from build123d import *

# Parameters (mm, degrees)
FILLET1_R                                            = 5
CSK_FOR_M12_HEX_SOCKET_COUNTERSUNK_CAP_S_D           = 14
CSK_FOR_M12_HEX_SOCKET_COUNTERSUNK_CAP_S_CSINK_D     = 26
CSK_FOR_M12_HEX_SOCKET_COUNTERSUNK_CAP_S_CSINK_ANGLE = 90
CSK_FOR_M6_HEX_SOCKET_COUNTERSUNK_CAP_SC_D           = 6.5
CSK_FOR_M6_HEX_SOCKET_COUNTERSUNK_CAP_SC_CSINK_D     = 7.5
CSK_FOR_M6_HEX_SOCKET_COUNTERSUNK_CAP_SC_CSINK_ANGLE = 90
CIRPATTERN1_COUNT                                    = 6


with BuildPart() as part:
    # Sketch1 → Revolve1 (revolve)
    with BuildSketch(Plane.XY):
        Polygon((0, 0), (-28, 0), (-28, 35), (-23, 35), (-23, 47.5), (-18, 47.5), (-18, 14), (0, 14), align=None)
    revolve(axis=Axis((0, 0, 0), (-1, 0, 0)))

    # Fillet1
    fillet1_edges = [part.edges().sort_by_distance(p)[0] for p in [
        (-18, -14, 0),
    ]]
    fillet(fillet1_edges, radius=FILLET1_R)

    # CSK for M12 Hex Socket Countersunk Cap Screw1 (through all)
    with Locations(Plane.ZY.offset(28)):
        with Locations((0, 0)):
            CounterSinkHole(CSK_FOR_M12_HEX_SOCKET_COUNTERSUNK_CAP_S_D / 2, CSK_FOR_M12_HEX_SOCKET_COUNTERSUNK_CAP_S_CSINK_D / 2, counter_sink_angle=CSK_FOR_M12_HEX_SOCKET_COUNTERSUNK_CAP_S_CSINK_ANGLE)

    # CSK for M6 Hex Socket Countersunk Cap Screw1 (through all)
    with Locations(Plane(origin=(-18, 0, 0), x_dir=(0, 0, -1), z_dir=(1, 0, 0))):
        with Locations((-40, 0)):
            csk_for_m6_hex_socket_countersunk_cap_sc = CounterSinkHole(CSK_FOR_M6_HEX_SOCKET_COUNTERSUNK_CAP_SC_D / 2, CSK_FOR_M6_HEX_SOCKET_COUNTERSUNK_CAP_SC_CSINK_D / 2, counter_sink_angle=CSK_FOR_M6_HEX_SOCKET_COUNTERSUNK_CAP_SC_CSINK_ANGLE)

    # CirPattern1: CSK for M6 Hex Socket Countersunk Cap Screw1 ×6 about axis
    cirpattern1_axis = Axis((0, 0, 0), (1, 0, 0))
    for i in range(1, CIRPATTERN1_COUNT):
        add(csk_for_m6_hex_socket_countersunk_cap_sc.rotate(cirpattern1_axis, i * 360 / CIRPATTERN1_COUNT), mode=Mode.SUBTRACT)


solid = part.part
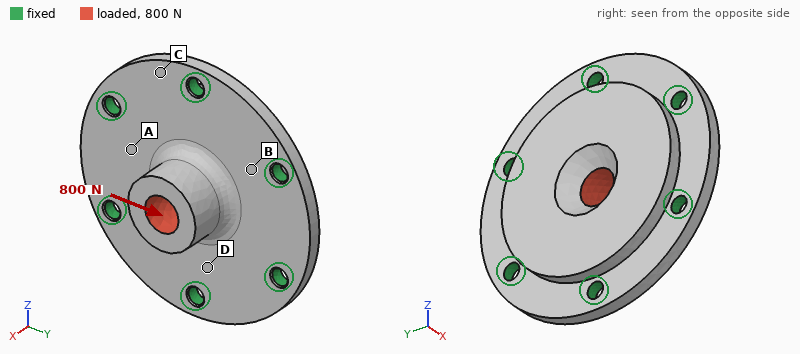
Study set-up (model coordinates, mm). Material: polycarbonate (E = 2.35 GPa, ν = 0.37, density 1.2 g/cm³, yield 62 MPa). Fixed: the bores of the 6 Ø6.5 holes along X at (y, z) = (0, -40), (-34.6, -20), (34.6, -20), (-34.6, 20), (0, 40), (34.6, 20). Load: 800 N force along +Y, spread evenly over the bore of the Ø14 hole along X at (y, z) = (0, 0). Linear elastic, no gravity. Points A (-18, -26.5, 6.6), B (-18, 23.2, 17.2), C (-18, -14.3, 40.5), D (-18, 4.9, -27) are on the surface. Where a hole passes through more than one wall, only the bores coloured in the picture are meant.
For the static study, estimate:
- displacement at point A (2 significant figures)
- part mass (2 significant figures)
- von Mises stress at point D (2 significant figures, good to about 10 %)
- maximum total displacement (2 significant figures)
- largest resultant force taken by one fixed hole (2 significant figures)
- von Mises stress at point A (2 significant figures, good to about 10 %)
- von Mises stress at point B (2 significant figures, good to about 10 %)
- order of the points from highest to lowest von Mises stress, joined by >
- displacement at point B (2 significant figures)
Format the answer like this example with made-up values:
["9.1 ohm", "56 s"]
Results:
["0.027 mm", "72 g", "1.2 MPa", "0.10 mm", "170 N", "1.9 MPa", "2.5 MPa", "B > A > D > C", "0.017 mm"]
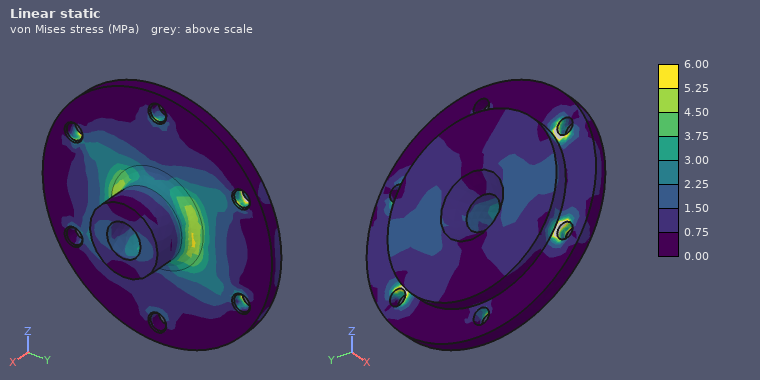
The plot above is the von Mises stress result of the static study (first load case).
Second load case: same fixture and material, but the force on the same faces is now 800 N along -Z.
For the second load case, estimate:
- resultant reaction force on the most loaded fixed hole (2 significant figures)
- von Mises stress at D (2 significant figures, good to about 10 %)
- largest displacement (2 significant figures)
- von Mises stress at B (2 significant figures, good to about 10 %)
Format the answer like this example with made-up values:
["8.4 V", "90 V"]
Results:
["190 N", "2.5 MPa", "0.10 mm", "1.3 MPa"]
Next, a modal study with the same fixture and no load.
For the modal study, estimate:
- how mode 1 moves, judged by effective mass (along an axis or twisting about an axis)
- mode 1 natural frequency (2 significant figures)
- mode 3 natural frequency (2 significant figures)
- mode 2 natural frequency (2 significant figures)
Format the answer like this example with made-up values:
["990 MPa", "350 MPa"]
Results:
["along X", "2400 Hz", "3600 Hz", "3600 Hz"]
